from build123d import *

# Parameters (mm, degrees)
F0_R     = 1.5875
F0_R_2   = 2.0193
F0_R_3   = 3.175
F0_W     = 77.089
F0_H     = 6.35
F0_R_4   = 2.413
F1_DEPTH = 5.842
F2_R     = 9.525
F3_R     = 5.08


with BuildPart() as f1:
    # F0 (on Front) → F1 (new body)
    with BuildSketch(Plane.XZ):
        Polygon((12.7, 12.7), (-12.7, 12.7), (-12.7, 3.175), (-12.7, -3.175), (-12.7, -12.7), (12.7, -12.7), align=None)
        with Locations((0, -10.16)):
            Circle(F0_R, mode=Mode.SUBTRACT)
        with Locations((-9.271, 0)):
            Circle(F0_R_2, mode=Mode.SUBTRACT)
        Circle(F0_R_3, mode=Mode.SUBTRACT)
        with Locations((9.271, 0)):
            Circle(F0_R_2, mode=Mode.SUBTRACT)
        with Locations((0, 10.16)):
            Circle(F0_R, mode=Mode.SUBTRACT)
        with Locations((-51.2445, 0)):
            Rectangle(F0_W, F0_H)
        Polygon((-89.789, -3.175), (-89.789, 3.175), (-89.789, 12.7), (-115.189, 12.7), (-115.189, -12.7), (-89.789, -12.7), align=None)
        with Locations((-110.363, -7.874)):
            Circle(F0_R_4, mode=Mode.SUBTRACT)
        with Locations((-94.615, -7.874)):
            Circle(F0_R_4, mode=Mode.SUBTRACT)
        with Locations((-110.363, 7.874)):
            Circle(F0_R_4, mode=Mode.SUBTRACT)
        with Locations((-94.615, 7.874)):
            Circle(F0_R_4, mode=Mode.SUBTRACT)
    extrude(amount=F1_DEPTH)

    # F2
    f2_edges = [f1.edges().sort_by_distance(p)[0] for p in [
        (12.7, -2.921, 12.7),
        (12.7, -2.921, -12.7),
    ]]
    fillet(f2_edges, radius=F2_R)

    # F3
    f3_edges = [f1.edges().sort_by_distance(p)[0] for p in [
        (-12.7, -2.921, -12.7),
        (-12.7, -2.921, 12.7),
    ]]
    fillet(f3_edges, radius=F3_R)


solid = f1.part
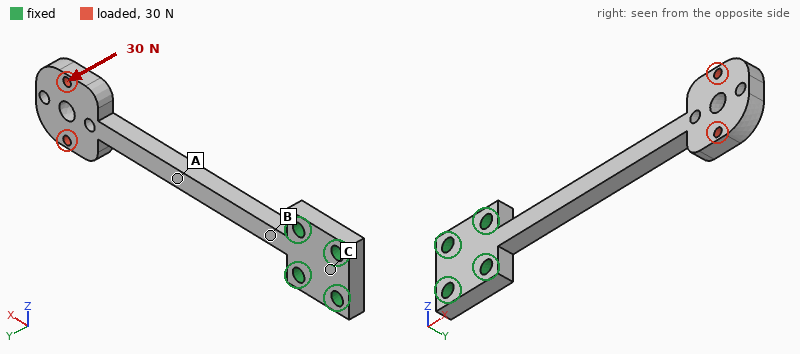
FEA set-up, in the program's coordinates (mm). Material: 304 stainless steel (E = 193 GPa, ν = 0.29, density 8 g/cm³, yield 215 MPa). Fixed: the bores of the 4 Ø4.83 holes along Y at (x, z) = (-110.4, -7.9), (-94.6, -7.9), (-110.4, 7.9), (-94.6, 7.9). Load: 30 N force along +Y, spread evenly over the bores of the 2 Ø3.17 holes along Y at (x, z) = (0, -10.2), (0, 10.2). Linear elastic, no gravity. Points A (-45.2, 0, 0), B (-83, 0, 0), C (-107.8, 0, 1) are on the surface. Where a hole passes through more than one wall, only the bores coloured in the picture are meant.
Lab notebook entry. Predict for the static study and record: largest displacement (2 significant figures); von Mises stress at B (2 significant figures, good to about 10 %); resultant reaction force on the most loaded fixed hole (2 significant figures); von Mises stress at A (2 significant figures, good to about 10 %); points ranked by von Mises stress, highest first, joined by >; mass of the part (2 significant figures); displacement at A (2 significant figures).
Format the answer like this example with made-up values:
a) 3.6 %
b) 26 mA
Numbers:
a) 0.48 mm
b) 69 MPa
c) 44 N
d) 38 MPa
e) B > A > C
f) 74 g
g) 0.13 mm
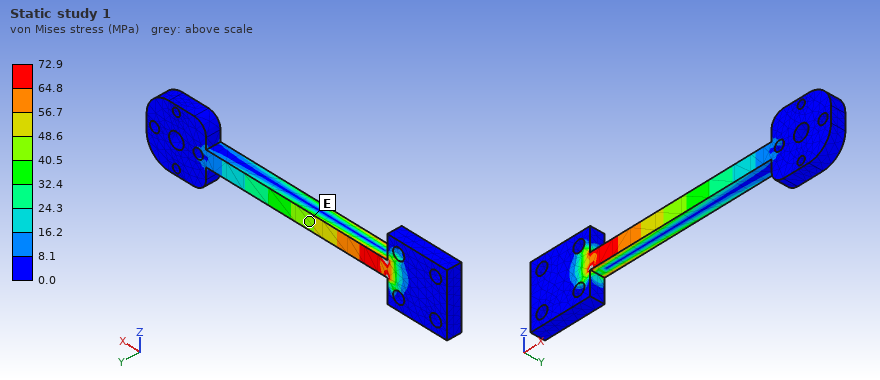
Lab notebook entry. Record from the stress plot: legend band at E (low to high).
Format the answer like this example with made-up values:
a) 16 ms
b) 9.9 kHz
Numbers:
a) 40.5 to 48.6 MPa
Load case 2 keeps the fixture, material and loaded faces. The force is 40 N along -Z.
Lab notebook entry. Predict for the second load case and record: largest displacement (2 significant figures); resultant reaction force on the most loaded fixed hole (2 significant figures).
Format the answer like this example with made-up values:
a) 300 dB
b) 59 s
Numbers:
a) 0.52 mm
b) 290 N
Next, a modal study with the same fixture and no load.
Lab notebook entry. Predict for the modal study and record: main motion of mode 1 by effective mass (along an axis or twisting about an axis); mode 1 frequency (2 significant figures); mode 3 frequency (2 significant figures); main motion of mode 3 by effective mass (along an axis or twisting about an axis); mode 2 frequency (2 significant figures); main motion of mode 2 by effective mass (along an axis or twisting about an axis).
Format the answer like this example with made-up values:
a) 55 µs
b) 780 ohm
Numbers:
a) along Y
b) 260 Hz
c) 1800 Hz
d) twisting about X
e) 290 Hz
f) along Z
